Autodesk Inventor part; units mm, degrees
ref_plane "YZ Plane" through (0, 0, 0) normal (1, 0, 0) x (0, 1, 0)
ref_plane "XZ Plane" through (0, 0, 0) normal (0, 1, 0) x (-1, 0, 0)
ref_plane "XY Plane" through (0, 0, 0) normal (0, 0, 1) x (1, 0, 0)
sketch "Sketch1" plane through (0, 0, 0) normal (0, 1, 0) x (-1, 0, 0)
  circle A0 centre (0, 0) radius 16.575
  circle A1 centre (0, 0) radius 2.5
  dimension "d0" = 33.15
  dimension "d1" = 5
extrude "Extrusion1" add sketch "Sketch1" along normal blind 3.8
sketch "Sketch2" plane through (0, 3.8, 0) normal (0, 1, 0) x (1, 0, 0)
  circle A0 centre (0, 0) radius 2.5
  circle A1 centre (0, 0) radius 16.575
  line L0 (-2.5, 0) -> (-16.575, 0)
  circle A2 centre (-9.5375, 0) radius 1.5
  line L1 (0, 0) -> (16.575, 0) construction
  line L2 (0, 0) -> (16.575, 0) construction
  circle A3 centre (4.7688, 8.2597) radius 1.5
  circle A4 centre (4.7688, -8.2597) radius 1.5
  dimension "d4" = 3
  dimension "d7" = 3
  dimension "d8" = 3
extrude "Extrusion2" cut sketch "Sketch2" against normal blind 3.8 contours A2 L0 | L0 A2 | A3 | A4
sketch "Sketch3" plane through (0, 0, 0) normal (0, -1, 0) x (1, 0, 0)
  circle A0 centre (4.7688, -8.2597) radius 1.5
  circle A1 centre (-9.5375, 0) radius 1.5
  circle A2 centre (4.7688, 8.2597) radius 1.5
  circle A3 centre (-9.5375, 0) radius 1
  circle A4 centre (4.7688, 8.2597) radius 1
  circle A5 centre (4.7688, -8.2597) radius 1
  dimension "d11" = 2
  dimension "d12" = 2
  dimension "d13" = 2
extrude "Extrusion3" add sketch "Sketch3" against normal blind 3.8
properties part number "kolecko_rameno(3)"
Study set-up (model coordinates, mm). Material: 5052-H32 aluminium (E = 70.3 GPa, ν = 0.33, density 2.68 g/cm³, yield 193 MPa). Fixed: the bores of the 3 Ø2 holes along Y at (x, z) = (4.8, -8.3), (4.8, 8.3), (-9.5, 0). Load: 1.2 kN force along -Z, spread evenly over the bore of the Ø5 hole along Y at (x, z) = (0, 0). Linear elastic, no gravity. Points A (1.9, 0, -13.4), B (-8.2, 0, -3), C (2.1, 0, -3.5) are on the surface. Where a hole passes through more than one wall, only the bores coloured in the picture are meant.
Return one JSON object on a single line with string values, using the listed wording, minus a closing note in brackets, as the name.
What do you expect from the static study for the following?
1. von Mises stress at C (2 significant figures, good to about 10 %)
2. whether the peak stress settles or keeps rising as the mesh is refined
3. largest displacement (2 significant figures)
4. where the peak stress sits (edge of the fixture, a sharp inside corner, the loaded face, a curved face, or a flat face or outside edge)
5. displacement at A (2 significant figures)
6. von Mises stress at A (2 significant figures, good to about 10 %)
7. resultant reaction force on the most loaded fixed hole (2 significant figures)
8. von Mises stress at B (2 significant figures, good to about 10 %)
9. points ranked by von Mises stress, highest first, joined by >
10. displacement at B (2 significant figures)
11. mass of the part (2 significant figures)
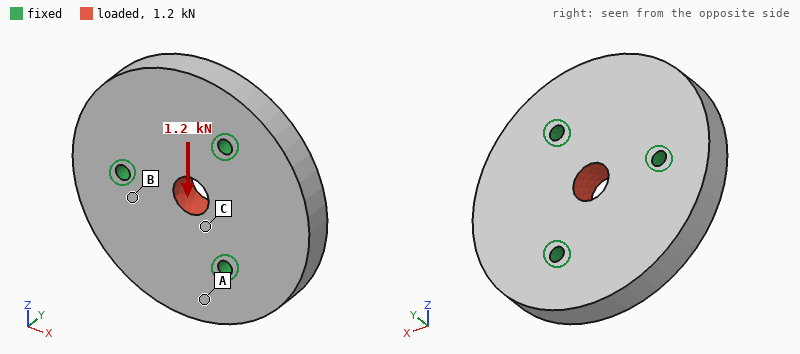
{"von Mises stress at C": "19 MPa", "whether the peak stress settles or keeps rising as the mesh is refined": "keeps rising", "largest displacement": "2.6 µm", "where the peak stress sits": "edge of the fixture", "displacement at A": "0.61 µm", "von Mises stress at A": "4.6 MPa", "resultant reaction force on the most loaded fixed hole": "420 N", "von Mises stress at B": "11 MPa", "points ranked by von Mises stress, highest first, joined by >": "C > B > A", "displacement at B": "0.63 µm", "mass of the part": "8.5 g"}
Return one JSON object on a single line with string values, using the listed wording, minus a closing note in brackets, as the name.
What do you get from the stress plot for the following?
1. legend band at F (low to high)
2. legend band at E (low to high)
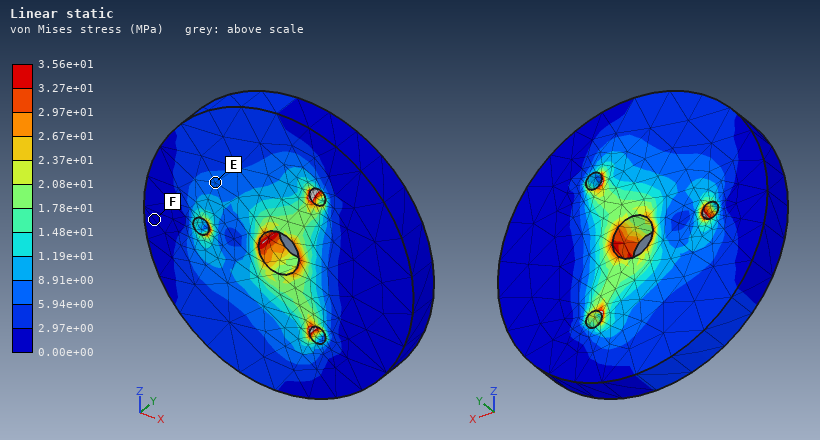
{"legend band at F": "0.00e+00 to 2.97e+00 MPa", "legend band at E": "5.94e+00 to 8.91e+00 MPa"}
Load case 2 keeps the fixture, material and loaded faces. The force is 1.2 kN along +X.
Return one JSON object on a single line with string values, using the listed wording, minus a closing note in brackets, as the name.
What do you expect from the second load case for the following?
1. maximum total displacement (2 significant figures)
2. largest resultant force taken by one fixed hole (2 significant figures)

{"maximum total displacement": "2.7 µm", "largest resultant force taken by one fixed hole": "430 N"}
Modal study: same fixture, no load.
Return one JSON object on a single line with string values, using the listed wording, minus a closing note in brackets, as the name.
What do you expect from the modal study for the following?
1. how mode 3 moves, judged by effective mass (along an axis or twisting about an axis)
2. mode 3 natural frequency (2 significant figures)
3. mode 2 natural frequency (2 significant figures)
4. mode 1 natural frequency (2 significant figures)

{"how mode 3 moves, judged by effective mass": "along Y", "mode 3 natural frequency": "25 kHz", "mode 2 natural frequency": "21 kHz", "mode 1 natural frequency": "21 kHz"}
